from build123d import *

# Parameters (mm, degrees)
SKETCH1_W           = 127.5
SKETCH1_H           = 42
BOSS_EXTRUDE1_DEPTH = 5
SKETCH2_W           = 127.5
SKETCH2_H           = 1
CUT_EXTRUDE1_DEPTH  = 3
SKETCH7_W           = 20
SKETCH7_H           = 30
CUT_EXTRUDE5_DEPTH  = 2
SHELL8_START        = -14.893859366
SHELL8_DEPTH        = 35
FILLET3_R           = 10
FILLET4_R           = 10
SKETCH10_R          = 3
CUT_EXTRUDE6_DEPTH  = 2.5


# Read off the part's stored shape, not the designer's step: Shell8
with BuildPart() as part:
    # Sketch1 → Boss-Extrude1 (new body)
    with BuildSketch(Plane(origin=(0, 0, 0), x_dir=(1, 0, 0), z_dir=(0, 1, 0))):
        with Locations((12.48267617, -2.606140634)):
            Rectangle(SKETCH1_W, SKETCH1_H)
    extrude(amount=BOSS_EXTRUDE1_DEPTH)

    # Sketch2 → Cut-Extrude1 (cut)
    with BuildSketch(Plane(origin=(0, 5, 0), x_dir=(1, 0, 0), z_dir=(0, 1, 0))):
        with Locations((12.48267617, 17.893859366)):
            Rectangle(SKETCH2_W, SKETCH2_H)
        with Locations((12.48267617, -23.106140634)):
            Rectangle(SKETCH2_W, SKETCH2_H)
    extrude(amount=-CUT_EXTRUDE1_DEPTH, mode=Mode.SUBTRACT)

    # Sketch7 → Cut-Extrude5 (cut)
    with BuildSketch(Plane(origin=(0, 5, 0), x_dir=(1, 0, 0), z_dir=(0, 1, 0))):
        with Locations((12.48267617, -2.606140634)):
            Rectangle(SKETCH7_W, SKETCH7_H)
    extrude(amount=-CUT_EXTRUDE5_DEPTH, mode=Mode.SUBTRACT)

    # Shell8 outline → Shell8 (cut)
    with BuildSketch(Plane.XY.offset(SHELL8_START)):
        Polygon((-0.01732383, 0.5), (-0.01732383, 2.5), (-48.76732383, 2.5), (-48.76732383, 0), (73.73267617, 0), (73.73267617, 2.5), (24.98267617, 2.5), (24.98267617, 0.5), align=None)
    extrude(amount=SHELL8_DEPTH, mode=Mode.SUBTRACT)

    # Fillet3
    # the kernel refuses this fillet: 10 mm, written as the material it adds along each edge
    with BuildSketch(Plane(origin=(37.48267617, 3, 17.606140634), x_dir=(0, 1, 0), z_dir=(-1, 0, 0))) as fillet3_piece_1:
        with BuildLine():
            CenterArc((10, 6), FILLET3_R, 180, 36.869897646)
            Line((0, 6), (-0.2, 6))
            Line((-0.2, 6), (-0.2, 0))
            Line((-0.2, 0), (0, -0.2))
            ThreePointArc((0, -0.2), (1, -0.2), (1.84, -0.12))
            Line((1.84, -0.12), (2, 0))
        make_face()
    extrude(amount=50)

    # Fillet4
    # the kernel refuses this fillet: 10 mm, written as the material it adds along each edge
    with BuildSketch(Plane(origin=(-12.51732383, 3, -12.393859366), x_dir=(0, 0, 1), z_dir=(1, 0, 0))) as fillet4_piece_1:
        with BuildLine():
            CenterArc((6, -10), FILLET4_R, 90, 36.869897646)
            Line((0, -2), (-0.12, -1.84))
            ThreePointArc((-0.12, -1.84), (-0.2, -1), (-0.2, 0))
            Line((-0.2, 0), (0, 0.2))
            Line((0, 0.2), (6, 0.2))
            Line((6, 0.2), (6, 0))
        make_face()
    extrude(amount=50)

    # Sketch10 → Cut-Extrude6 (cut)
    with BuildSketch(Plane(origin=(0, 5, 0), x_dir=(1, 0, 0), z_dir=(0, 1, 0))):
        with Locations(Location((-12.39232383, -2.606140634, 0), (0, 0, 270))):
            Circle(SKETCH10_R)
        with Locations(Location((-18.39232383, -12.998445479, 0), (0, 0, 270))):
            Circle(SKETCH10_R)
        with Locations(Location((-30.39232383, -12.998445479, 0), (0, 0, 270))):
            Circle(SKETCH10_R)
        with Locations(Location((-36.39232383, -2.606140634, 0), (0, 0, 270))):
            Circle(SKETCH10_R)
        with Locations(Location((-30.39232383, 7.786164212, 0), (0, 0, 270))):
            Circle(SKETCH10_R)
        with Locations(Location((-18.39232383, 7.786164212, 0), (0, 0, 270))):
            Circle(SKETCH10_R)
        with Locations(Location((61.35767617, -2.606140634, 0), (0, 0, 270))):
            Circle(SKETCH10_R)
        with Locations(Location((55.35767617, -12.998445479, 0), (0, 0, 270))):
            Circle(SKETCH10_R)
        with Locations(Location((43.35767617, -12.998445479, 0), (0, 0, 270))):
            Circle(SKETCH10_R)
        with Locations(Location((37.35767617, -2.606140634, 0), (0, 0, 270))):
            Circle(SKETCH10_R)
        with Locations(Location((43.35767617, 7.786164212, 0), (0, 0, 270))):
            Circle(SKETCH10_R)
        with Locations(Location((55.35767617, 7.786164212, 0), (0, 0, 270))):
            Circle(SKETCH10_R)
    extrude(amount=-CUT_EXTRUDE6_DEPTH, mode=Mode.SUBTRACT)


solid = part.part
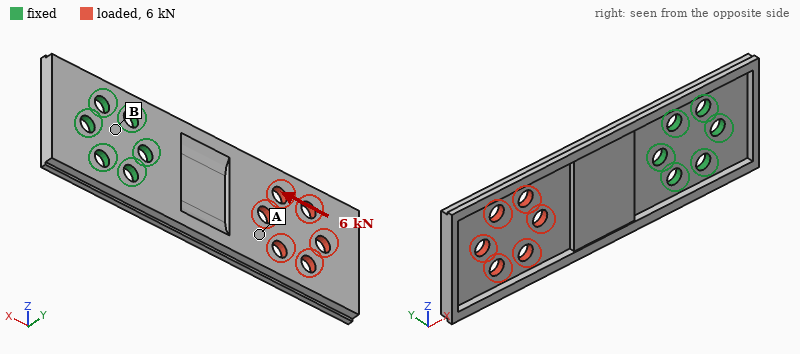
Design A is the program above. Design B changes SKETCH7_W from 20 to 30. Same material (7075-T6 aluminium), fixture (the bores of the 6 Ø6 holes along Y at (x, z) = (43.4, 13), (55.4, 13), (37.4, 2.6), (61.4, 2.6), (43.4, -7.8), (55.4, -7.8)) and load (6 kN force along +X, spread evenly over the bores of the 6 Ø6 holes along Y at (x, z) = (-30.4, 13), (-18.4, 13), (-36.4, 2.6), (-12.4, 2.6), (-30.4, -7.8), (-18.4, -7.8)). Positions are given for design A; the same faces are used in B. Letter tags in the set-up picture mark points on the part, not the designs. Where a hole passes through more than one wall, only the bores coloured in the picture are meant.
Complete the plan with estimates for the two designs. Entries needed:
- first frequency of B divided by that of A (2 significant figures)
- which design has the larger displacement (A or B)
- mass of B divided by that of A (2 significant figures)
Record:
0.91
B
0.97
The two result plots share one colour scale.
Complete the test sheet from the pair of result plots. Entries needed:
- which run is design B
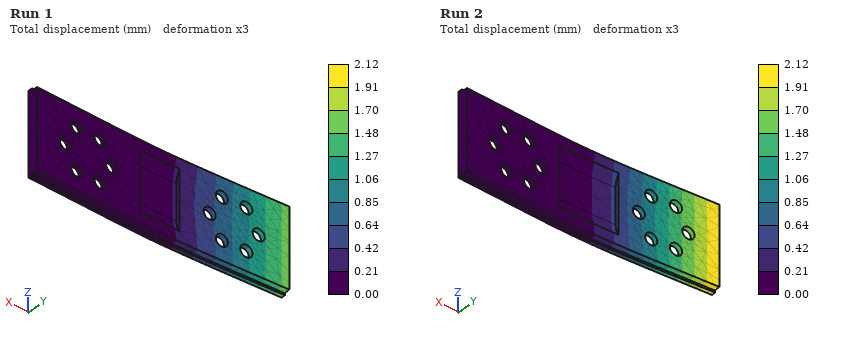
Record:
Run 2
